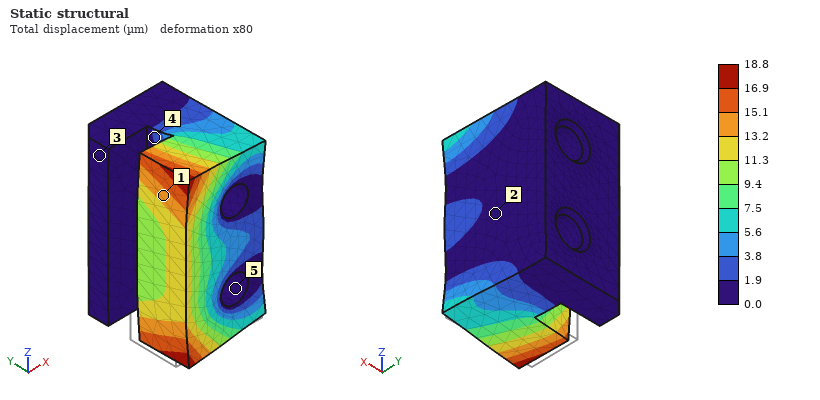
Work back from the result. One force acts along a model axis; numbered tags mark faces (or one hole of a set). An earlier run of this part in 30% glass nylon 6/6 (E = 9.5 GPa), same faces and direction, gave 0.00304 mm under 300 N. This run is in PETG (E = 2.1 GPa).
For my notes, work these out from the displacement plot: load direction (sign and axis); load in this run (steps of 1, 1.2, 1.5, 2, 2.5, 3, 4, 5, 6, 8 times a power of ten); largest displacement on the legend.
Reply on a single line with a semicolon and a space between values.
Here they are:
+X; 400 N; 18.8 µm
